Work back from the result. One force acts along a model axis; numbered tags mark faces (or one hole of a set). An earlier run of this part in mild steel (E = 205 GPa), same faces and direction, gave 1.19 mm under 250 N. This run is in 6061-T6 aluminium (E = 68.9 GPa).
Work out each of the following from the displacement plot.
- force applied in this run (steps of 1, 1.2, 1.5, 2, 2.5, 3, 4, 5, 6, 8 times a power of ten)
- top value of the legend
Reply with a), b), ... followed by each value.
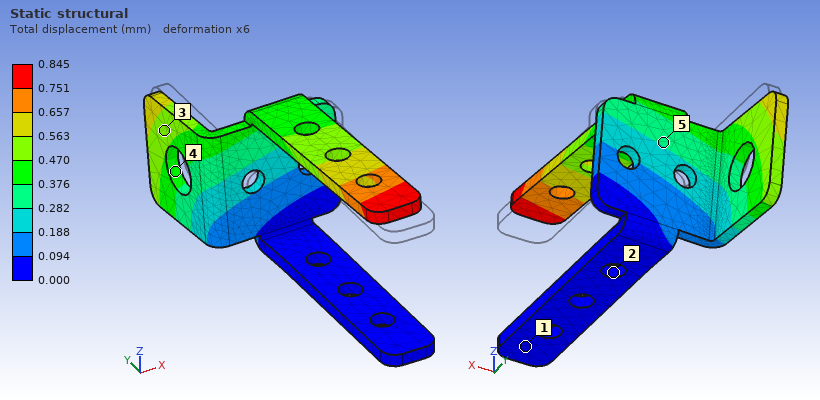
a) 60 N
b) 0.845 mm
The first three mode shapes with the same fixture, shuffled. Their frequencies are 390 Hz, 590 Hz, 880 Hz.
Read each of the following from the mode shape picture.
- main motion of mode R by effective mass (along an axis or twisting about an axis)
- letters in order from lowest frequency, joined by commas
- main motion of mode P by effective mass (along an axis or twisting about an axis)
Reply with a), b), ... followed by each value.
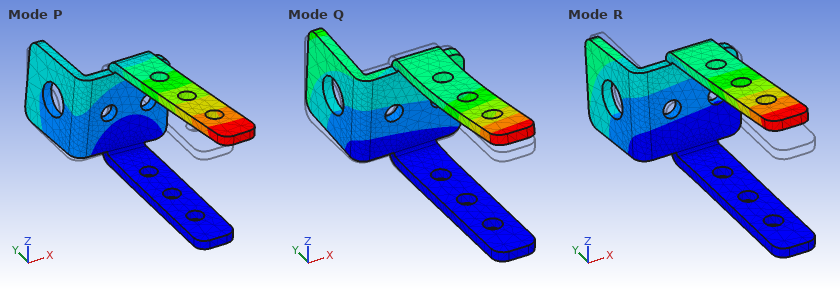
a) along Y
b) R, P, Q
c) along X
